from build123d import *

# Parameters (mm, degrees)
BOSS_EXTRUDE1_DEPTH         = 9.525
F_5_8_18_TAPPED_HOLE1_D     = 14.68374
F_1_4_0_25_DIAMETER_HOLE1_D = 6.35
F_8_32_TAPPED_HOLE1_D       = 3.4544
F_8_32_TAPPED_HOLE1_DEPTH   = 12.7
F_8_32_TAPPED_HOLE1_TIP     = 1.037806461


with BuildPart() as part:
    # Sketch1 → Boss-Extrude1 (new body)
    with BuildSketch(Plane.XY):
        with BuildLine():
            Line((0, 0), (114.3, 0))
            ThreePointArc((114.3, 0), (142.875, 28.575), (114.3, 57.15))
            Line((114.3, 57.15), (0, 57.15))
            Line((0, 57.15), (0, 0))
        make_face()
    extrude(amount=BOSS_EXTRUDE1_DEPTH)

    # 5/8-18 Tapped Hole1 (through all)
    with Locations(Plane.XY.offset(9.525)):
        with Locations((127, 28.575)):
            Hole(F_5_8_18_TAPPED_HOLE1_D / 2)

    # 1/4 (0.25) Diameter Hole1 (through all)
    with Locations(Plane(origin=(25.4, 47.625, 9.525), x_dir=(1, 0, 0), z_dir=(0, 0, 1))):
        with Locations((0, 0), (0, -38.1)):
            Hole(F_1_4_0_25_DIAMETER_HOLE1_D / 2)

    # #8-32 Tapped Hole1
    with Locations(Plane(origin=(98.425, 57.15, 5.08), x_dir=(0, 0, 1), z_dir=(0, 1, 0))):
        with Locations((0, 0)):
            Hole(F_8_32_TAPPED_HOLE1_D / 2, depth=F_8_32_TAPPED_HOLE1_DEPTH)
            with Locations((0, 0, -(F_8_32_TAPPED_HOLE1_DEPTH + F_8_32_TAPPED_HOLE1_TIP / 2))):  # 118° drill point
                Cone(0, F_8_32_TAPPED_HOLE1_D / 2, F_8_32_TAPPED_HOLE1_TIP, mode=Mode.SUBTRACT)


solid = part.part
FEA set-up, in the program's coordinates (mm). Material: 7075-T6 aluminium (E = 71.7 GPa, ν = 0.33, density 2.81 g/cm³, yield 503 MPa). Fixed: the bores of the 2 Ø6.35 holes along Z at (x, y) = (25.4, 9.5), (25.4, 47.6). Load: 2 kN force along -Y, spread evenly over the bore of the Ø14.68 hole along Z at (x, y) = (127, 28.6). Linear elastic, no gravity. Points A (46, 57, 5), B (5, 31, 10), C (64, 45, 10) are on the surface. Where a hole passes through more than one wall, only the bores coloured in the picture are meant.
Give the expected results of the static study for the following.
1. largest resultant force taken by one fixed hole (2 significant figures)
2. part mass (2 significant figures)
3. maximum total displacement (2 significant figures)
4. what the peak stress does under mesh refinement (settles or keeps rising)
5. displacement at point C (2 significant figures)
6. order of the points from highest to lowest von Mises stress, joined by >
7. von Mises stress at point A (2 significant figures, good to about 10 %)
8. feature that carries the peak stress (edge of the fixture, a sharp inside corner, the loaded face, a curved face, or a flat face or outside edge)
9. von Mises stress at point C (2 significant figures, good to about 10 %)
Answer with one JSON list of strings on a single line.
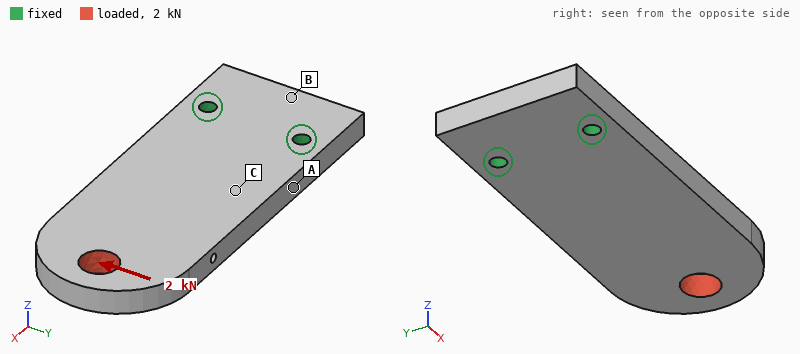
["5.1 kN", "200 g", "0.10 mm", "keeps rising", "0.023 mm", "A > C > B", "30 MPa", "edge of the fixture", "15 MPa"]
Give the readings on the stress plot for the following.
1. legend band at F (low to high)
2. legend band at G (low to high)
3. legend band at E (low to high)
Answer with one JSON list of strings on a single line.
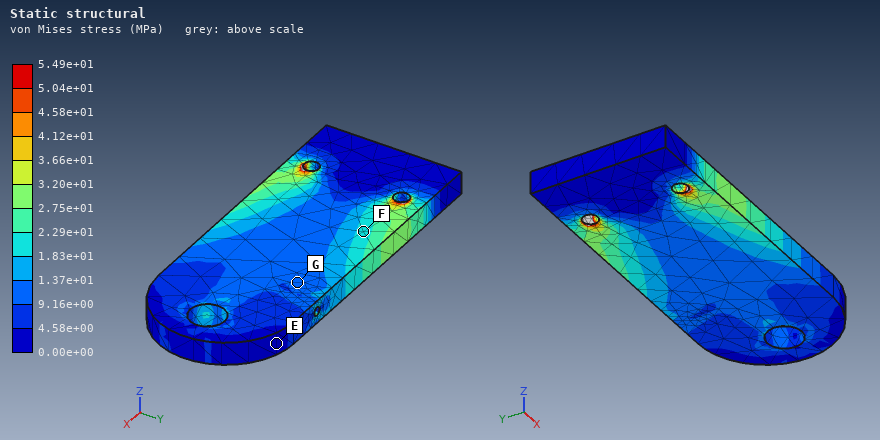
["1.83e+01 to 2.29e+01 MPa", "9.16e+00 to 1.37e+01 MPa", "0.00e+00 to 4.58e+00 MPa"]
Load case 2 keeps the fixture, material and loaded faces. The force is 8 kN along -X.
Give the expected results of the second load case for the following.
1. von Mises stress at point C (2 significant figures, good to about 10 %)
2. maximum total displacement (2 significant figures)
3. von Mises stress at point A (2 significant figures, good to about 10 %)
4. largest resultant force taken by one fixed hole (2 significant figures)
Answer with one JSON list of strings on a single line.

["15 MPa", "32 µm", "15 MPa", "4.0 kN"]
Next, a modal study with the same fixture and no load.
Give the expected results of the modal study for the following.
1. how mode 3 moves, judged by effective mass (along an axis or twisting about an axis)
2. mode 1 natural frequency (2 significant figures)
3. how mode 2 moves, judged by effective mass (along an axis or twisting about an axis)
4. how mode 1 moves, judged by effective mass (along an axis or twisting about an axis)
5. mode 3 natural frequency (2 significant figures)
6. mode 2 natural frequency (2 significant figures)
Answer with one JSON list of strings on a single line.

["along Y", "640 Hz", "twisting about X", "along Z", "3200 Hz", "2600 Hz"]
